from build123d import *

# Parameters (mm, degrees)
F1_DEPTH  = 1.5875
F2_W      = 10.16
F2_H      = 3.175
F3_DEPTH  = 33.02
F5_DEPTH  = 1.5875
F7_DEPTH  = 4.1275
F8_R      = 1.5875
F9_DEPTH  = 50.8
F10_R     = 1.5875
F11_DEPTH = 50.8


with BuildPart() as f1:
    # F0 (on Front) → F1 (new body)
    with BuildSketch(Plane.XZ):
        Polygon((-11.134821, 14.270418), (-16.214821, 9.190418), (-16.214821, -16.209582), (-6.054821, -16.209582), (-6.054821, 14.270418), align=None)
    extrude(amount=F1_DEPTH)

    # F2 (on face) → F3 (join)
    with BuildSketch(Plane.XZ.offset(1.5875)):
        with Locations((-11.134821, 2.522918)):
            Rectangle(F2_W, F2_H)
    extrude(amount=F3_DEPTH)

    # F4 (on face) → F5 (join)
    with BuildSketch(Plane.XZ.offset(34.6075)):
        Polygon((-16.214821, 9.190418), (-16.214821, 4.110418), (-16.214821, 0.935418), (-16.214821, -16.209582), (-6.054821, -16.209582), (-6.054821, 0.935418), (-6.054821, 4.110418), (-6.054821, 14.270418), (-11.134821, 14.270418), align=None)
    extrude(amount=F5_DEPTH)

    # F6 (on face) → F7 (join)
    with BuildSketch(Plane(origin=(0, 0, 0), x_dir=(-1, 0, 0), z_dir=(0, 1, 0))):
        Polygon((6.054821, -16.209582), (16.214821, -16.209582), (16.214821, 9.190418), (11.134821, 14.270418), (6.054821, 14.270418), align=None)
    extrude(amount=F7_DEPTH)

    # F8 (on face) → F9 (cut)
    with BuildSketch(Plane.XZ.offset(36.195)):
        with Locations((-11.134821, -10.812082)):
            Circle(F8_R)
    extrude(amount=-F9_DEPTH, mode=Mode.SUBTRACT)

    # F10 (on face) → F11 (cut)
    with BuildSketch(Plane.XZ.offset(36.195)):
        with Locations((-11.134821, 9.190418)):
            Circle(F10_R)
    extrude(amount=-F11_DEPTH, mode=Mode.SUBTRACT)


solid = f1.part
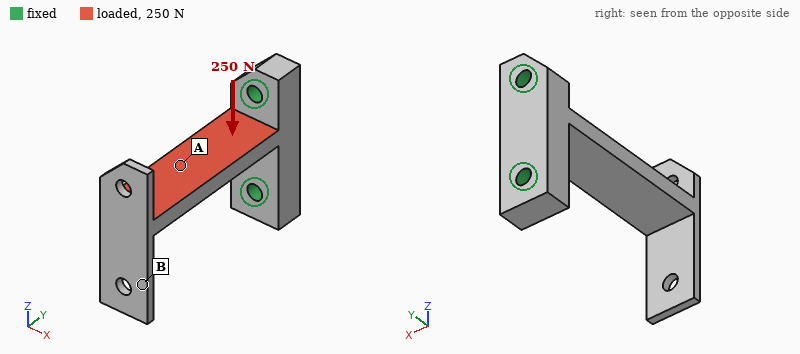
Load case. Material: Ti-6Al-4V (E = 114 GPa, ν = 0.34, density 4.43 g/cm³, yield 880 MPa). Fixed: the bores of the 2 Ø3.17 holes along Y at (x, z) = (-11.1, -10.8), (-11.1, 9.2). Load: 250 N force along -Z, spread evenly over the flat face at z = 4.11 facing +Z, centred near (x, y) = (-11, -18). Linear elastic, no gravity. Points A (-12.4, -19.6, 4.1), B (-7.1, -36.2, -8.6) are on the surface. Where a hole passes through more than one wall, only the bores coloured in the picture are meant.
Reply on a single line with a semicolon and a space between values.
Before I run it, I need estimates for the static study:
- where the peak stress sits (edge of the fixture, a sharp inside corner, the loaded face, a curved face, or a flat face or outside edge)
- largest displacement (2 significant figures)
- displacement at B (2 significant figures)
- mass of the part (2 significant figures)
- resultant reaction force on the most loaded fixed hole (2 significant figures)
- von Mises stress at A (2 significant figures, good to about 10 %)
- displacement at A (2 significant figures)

the loaded face; 0.54 mm; 0.48 mm; 14 g; 340 N; 51 MPa; 0.18 mm
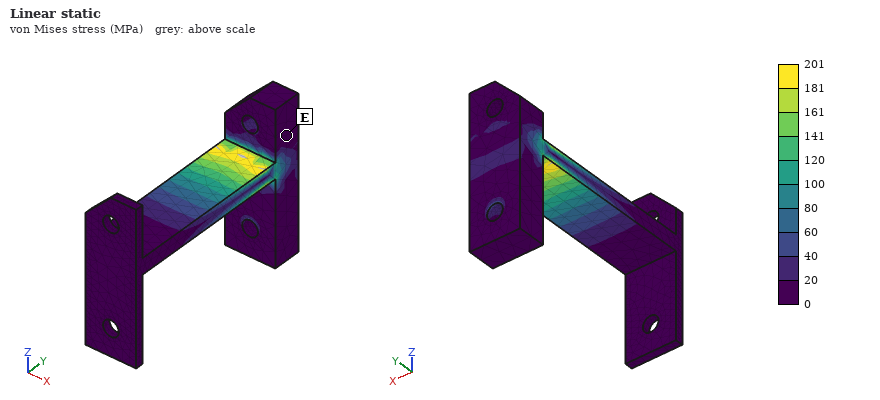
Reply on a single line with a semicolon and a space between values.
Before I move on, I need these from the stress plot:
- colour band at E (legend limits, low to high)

0 to 20 MPa
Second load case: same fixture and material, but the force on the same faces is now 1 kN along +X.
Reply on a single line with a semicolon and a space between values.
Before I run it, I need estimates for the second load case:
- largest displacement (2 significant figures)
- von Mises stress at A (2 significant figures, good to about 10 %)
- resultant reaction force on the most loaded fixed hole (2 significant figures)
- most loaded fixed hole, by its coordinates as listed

0.42 mm; 82 MPa; 810 N; (-11.1, 9.2)
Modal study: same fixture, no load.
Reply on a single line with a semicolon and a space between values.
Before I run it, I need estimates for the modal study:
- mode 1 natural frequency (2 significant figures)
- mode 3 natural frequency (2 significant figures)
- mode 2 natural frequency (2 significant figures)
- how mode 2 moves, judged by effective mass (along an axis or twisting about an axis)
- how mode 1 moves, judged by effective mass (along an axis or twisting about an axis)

1300 Hz; 3800 Hz; 3000 Hz; along X; along Z
